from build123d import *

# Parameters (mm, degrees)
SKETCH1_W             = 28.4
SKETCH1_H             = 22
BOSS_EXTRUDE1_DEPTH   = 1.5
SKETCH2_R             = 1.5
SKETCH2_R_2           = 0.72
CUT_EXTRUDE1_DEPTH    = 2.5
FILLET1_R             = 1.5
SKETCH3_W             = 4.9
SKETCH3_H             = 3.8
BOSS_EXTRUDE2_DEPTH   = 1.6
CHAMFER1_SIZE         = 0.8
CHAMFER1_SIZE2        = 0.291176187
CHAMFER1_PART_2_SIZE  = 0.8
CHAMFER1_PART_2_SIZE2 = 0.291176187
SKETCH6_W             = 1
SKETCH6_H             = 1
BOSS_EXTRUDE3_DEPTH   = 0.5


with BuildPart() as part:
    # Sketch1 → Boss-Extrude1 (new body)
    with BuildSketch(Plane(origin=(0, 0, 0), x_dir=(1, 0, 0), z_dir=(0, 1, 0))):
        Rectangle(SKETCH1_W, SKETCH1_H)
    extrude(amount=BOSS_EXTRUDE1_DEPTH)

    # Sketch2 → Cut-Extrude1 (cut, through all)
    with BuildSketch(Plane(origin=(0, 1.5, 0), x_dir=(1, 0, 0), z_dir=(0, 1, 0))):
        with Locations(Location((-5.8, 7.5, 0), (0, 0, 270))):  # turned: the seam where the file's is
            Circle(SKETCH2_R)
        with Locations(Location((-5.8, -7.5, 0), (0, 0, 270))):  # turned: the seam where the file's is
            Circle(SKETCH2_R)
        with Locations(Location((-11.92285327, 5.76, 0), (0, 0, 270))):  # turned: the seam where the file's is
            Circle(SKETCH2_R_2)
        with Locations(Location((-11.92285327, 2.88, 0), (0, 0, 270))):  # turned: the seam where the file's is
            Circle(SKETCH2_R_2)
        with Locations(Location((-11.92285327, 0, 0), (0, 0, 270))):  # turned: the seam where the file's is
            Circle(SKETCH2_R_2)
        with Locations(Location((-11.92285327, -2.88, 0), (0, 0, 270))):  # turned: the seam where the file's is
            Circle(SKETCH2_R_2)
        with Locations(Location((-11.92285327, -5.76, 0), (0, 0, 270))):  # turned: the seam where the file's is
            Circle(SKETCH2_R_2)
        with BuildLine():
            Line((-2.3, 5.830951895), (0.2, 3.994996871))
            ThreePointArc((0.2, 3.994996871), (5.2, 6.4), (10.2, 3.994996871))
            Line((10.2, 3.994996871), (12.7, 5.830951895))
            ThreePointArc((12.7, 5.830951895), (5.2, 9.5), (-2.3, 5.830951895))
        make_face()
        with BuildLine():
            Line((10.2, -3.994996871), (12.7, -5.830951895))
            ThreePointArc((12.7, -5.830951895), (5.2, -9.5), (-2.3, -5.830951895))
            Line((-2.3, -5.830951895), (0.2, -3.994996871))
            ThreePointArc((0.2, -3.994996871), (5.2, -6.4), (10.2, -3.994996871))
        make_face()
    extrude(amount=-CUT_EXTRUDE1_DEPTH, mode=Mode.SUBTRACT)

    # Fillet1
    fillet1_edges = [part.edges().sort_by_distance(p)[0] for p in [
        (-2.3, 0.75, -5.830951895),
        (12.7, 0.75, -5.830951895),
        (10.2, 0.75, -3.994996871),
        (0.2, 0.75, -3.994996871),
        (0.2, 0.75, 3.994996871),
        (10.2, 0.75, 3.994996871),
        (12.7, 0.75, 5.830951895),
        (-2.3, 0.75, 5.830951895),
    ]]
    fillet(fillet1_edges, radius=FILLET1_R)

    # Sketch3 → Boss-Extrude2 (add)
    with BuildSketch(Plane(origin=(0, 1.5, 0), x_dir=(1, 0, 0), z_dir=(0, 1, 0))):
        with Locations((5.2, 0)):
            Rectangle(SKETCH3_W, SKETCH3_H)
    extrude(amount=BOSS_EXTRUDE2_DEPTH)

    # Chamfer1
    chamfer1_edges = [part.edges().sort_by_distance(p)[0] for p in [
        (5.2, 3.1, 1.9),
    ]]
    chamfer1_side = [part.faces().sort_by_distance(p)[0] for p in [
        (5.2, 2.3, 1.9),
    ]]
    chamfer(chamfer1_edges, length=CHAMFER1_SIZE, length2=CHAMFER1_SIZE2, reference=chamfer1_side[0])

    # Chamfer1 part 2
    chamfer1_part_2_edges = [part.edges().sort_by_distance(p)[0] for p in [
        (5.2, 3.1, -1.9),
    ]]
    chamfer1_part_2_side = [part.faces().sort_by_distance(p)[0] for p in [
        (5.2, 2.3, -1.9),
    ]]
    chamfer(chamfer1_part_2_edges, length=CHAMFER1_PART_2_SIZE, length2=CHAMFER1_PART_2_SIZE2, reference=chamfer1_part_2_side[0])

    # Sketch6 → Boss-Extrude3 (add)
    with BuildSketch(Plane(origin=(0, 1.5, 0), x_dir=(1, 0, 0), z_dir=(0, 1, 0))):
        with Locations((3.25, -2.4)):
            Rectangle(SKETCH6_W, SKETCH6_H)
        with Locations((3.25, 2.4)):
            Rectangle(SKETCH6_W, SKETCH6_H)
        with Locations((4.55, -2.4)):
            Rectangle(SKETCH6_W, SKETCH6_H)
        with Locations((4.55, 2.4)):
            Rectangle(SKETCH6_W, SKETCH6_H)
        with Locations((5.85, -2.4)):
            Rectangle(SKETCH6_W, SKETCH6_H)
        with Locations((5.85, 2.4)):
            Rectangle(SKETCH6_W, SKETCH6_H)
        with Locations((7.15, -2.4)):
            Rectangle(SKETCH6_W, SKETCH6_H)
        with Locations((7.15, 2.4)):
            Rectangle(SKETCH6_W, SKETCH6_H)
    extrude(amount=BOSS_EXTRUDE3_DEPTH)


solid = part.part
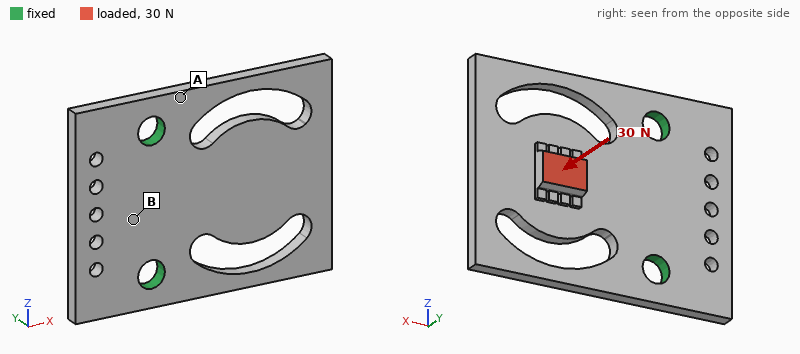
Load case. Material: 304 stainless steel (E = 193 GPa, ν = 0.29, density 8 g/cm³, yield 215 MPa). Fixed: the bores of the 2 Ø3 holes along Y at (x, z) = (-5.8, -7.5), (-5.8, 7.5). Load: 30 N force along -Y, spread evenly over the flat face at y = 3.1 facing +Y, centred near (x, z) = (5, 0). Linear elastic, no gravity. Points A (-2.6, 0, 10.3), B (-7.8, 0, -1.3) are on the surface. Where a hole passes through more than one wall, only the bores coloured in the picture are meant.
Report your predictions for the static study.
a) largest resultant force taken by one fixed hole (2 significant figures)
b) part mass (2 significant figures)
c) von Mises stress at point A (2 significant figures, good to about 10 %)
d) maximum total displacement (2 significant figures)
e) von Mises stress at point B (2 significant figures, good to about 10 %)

15 N
6.5 g
25 MPa
32 µm
8.5 MPa
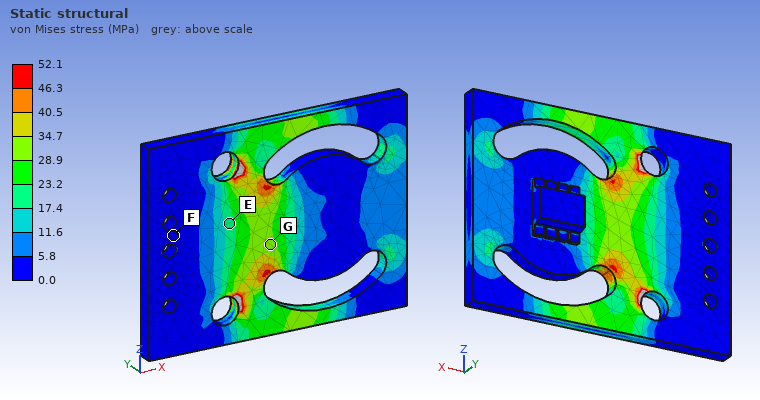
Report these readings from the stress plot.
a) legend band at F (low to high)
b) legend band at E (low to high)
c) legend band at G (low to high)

0.0 to 5.8 MPa
17.4 to 23.2 MPa
28.9 to 34.7 MPa
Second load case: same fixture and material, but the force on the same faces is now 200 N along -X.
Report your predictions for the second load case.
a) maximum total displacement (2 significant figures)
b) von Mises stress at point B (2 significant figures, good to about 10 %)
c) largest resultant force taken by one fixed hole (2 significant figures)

76 µm
10 MPa
100 N
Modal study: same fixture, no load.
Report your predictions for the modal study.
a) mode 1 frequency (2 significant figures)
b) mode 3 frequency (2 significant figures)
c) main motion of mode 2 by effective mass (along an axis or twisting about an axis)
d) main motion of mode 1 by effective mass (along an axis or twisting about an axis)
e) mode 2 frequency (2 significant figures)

3000 Hz
13 kHz
twisting about X
along Y
7200 Hz
